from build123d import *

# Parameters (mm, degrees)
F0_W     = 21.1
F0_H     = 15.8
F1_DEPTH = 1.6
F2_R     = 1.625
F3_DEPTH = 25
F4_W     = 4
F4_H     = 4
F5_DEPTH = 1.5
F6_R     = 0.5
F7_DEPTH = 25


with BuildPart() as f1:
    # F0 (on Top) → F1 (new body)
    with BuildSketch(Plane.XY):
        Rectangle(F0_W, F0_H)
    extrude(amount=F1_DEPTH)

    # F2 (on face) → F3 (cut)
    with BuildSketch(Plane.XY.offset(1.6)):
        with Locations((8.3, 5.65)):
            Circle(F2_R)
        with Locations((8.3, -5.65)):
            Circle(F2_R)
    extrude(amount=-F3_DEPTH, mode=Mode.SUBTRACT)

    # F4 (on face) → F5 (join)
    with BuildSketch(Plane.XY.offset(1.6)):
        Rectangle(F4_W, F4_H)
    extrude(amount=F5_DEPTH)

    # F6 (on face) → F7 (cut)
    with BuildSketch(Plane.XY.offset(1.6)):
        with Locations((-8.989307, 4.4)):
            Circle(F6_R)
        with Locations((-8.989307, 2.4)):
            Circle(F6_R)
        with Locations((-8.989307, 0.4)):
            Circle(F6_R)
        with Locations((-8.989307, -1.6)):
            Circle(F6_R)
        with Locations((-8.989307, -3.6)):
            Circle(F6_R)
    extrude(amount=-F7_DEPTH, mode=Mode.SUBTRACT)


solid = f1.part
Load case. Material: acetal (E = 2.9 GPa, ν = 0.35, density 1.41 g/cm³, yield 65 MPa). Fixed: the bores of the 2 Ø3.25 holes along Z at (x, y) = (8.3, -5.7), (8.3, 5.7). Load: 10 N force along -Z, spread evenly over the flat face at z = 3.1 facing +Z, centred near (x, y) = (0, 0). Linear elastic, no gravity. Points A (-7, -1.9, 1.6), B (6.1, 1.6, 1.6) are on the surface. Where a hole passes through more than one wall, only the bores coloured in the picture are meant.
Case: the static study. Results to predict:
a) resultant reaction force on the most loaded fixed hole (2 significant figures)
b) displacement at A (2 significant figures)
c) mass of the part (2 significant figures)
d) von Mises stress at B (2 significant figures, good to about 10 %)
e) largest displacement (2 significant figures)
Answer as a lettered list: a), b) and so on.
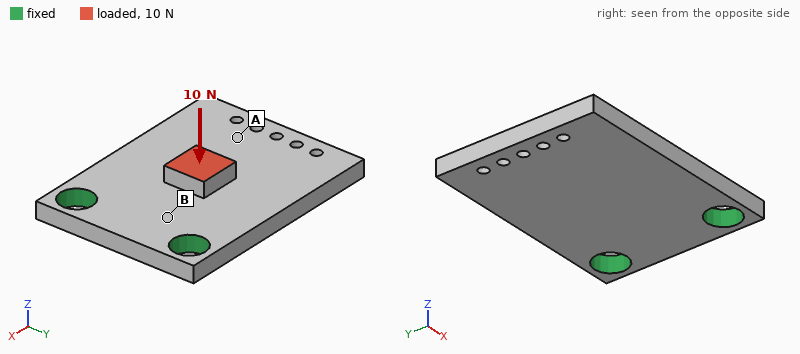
a) 5.0 N
b) 0.22 mm
c) 0.74 g
d) 5.8 MPa
e) 0.28 mm
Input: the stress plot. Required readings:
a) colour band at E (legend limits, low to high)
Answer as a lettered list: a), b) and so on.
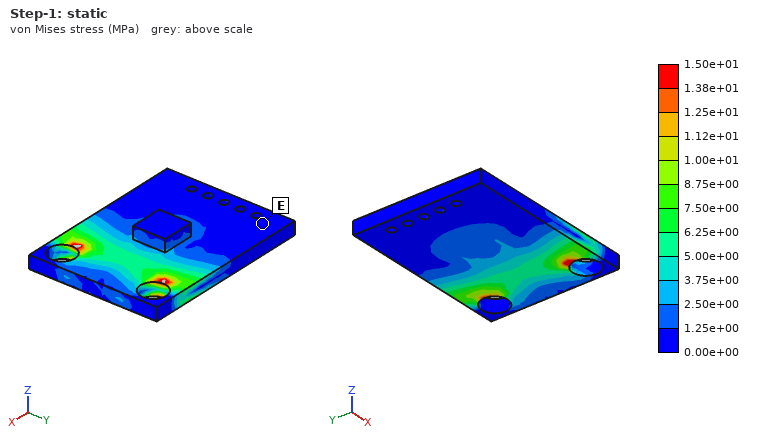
a) 0.00e+00 to 1.25e+00 MPa
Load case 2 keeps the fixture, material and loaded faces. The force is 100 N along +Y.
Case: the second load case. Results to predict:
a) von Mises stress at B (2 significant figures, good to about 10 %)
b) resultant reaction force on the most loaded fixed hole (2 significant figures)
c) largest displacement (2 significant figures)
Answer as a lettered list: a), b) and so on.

a) 15 MPa
b) 82 N
c) 0.29 mm
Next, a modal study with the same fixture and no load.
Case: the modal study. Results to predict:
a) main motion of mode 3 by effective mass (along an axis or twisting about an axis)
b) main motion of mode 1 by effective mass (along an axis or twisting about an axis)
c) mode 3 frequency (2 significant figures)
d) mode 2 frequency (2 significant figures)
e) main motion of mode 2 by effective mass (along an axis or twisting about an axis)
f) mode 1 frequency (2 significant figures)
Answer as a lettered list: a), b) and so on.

a) along Z
b) along Z
c) 7100 Hz
d) 3300 Hz
e) twisting about X
f) 1200 Hz
